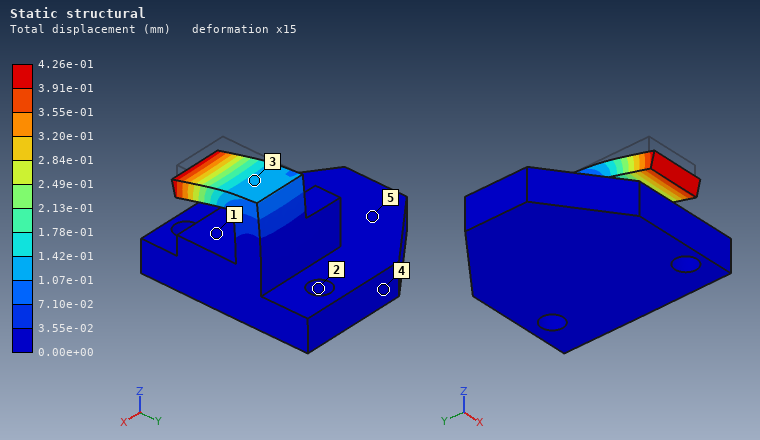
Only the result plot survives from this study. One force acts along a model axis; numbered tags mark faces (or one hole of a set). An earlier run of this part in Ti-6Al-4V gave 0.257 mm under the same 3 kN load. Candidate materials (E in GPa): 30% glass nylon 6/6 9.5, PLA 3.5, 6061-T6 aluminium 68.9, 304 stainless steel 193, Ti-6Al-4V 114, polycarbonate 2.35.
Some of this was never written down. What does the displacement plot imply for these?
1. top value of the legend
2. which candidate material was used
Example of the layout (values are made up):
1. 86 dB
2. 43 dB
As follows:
1. 4.26e-01 mm
2. 6061-T6 aluminium
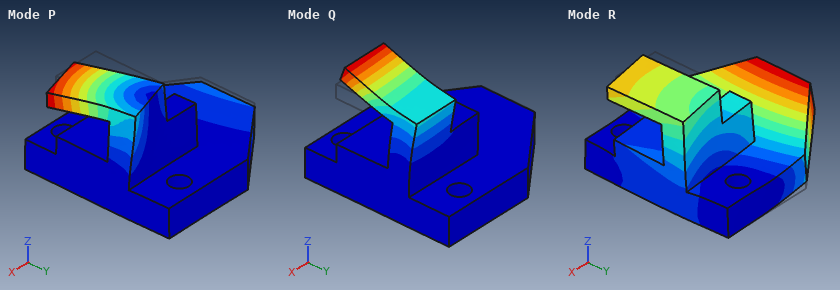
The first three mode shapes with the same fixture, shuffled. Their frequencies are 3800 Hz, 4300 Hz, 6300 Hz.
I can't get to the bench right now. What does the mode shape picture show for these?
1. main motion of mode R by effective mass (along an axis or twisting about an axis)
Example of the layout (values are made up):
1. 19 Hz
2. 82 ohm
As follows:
1. along Z
